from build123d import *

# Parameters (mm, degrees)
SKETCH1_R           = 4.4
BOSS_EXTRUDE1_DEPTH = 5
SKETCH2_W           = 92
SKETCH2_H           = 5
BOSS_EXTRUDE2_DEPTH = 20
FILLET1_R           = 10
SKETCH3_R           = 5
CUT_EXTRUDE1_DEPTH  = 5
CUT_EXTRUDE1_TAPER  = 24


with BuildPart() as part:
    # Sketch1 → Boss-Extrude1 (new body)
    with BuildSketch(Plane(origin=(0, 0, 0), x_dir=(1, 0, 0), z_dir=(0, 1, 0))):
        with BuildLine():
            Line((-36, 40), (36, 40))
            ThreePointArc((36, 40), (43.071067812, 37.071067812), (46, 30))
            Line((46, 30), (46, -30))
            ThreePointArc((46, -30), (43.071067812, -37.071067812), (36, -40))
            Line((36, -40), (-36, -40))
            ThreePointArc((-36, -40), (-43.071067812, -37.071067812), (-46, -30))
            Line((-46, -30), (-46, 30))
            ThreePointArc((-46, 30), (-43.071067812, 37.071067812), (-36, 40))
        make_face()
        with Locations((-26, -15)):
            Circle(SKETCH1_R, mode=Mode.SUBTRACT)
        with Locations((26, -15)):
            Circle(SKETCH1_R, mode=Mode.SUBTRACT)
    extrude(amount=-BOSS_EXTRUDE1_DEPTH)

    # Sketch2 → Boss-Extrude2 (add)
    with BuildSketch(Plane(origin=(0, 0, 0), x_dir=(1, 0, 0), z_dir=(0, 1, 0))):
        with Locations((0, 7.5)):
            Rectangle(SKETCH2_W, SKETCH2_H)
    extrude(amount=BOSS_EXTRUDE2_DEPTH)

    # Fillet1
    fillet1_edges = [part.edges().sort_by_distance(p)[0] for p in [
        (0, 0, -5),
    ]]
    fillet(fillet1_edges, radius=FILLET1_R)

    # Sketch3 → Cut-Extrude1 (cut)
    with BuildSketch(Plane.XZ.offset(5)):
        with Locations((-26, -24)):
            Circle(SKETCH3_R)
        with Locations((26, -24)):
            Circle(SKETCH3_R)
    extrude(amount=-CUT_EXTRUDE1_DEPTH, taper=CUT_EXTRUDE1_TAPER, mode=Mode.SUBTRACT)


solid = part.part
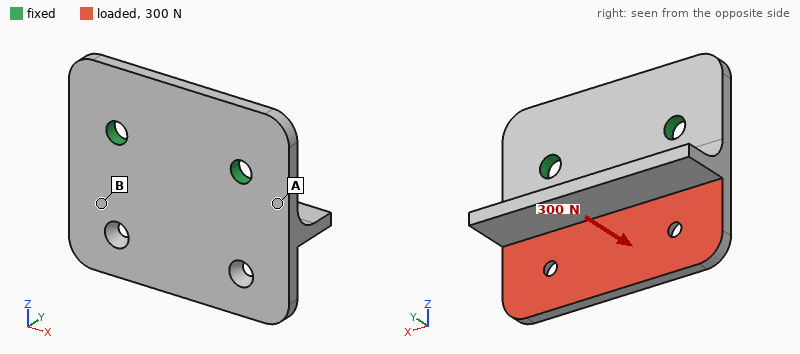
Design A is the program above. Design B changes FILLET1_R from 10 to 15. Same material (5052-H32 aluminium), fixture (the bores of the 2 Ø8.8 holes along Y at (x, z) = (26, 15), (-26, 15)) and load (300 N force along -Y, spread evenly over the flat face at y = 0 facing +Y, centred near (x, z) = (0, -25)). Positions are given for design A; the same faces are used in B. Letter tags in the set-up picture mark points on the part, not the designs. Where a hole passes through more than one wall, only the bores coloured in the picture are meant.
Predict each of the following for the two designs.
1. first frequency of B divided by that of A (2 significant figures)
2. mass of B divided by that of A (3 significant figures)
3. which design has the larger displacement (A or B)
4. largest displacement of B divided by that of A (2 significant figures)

1.1
1.05
A
0.86
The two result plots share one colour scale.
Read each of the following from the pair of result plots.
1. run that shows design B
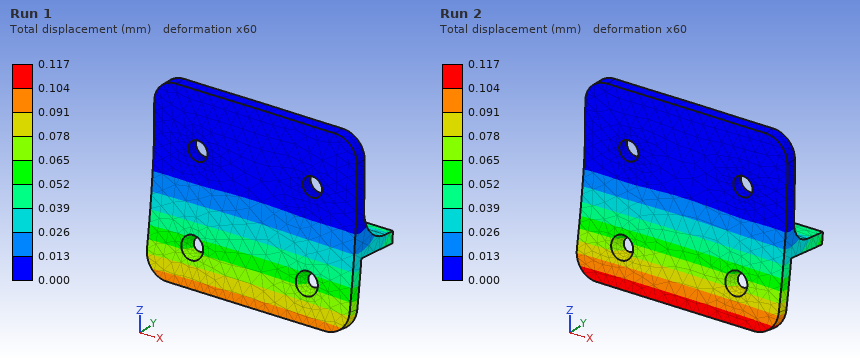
Run 1
